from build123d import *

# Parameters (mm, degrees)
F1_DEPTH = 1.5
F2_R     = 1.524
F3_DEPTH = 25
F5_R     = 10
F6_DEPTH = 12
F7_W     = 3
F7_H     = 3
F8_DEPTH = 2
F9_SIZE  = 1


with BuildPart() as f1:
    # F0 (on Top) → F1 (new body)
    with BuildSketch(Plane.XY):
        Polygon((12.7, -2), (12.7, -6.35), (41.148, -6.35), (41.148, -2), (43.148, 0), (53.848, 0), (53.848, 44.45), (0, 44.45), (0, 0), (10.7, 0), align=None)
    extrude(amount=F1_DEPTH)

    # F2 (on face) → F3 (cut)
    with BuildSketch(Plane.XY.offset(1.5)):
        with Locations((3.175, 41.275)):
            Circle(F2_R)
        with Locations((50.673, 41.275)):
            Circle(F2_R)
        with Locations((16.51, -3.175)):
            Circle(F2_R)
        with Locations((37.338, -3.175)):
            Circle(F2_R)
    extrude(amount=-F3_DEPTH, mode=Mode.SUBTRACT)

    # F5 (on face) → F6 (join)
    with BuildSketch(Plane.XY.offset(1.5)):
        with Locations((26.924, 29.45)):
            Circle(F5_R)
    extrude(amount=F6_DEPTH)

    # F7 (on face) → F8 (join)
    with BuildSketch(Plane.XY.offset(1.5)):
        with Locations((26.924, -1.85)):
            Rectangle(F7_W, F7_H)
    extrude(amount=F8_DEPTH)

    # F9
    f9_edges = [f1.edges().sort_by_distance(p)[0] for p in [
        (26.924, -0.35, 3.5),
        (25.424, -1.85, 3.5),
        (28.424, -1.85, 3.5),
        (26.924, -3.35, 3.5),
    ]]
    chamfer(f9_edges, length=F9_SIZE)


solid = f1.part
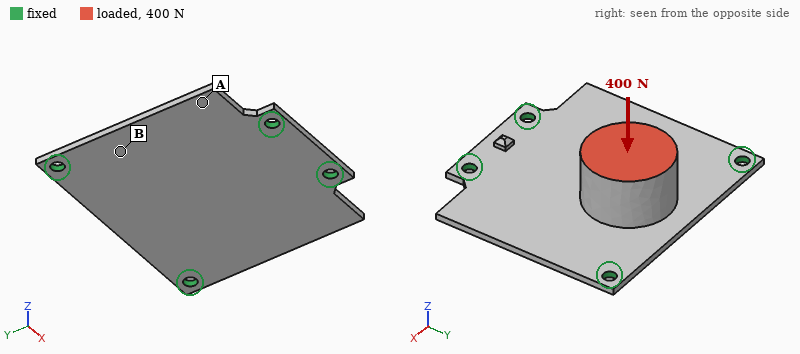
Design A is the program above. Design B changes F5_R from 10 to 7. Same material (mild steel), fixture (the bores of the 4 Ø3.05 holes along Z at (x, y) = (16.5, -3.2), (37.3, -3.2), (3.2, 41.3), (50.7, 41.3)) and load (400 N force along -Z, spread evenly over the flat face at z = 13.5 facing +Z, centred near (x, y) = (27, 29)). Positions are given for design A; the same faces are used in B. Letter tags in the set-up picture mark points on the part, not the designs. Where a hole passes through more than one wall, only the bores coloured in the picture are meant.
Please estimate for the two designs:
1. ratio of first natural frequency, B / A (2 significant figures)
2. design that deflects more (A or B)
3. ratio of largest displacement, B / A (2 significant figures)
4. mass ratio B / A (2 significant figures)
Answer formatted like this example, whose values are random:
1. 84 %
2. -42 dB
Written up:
1. 1.1
2. B
3. 1.5
4. 0.75
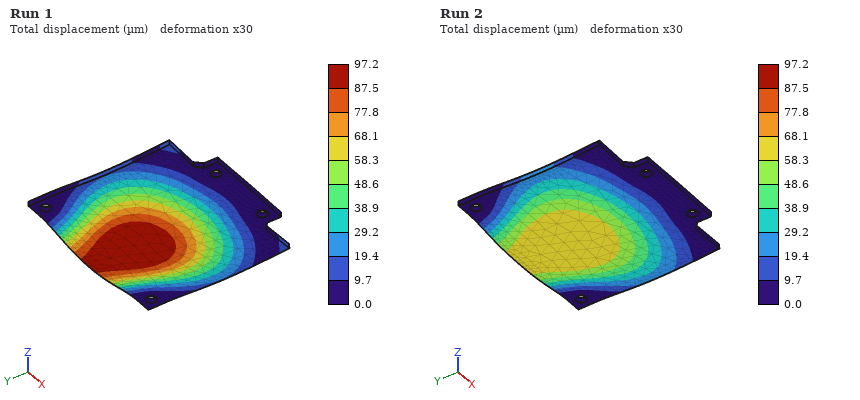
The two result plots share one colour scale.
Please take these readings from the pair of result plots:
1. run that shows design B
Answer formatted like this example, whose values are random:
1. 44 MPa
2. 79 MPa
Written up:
1. Run 1
